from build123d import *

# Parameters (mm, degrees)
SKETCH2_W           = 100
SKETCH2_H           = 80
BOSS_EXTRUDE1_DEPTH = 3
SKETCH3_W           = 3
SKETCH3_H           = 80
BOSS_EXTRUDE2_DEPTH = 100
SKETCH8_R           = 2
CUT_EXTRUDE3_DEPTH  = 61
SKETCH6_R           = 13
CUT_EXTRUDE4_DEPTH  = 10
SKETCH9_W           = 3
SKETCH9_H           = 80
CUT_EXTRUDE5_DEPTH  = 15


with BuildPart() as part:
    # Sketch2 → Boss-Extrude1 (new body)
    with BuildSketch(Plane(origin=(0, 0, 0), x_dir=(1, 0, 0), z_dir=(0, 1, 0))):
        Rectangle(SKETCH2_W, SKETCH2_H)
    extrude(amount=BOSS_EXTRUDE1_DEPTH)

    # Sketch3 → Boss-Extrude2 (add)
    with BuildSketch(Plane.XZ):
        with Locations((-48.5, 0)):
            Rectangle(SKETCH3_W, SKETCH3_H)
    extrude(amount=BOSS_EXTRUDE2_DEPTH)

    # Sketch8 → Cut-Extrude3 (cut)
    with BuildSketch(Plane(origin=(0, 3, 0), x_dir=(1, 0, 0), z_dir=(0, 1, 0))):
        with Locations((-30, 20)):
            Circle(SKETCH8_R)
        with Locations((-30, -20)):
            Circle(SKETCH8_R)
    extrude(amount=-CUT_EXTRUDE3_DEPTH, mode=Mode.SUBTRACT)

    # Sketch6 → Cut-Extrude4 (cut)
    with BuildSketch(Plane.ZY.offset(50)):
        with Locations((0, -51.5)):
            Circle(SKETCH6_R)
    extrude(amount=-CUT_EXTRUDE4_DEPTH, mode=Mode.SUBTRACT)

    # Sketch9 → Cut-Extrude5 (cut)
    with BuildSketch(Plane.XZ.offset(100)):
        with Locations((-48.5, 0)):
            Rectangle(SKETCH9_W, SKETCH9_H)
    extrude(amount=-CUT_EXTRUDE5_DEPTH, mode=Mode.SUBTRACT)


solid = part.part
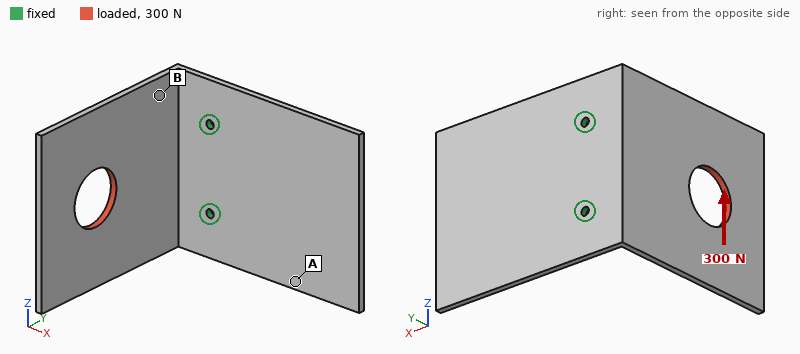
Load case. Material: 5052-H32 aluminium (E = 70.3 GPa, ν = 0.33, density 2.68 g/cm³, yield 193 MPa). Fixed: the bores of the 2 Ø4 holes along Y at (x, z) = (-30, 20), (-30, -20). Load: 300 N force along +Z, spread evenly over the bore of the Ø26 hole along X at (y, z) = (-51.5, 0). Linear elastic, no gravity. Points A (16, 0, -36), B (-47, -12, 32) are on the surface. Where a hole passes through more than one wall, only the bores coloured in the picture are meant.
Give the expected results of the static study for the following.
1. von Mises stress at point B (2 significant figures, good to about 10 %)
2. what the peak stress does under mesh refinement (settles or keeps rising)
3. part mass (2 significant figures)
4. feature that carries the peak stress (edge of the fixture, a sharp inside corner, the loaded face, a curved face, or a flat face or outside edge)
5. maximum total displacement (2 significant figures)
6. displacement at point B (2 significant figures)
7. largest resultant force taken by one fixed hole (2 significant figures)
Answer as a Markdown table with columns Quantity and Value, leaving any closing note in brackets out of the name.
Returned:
| Quantity | Value |
|---|---|
| von Mises stress at point B | 24 MPa |
| what the peak stress does under mesh refinement | keeps rising |
| part mass | 110 g |
| feature that carries the peak stress | edge of the fixture |
| maximum total displacement | 0.40 mm |
| displacement at point B | 0.14 mm |
| largest resultant force taken by one fixed hole | 400 N |
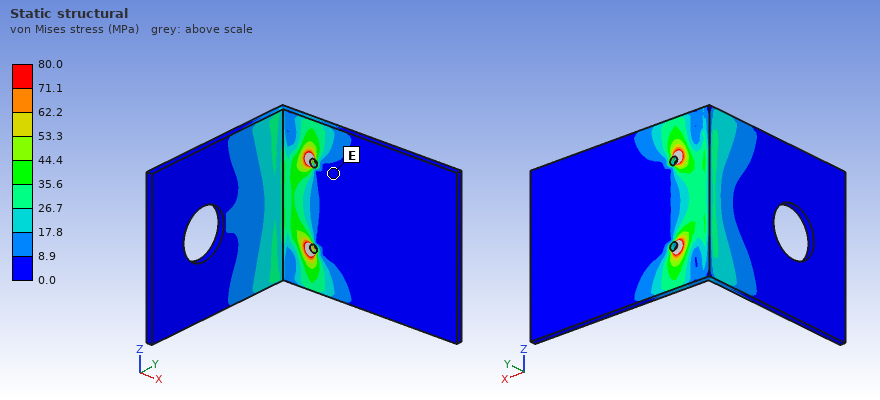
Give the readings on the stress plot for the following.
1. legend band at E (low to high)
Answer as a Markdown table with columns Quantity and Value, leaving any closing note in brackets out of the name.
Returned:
| Quantity | Value |
|---|---|
| legend band at E | 0.0 to 8.9 MPa |
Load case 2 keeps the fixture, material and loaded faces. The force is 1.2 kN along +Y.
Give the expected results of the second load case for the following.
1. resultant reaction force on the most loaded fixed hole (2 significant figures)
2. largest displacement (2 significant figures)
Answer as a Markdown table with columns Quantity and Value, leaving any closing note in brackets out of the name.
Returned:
| Quantity | Value |
|---|---|
| resultant reaction force on the most loaded fixed hole | 600 N |
| largest displacement | 1.7 mm |
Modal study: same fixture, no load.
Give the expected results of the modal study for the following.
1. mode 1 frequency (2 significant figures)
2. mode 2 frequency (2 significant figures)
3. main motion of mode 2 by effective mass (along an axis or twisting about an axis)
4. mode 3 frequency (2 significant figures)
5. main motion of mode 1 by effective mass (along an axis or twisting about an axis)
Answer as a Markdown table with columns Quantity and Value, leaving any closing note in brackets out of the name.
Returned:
| Quantity | Value |
|---|---|
| mode 1 frequency | 250 Hz |
| mode 2 frequency | 380 Hz |
| main motion of mode 2 by effective mass | along Y |
| mode 3 frequency | 670 Hz |
| main motion of mode 1 by effective mass | along X |
